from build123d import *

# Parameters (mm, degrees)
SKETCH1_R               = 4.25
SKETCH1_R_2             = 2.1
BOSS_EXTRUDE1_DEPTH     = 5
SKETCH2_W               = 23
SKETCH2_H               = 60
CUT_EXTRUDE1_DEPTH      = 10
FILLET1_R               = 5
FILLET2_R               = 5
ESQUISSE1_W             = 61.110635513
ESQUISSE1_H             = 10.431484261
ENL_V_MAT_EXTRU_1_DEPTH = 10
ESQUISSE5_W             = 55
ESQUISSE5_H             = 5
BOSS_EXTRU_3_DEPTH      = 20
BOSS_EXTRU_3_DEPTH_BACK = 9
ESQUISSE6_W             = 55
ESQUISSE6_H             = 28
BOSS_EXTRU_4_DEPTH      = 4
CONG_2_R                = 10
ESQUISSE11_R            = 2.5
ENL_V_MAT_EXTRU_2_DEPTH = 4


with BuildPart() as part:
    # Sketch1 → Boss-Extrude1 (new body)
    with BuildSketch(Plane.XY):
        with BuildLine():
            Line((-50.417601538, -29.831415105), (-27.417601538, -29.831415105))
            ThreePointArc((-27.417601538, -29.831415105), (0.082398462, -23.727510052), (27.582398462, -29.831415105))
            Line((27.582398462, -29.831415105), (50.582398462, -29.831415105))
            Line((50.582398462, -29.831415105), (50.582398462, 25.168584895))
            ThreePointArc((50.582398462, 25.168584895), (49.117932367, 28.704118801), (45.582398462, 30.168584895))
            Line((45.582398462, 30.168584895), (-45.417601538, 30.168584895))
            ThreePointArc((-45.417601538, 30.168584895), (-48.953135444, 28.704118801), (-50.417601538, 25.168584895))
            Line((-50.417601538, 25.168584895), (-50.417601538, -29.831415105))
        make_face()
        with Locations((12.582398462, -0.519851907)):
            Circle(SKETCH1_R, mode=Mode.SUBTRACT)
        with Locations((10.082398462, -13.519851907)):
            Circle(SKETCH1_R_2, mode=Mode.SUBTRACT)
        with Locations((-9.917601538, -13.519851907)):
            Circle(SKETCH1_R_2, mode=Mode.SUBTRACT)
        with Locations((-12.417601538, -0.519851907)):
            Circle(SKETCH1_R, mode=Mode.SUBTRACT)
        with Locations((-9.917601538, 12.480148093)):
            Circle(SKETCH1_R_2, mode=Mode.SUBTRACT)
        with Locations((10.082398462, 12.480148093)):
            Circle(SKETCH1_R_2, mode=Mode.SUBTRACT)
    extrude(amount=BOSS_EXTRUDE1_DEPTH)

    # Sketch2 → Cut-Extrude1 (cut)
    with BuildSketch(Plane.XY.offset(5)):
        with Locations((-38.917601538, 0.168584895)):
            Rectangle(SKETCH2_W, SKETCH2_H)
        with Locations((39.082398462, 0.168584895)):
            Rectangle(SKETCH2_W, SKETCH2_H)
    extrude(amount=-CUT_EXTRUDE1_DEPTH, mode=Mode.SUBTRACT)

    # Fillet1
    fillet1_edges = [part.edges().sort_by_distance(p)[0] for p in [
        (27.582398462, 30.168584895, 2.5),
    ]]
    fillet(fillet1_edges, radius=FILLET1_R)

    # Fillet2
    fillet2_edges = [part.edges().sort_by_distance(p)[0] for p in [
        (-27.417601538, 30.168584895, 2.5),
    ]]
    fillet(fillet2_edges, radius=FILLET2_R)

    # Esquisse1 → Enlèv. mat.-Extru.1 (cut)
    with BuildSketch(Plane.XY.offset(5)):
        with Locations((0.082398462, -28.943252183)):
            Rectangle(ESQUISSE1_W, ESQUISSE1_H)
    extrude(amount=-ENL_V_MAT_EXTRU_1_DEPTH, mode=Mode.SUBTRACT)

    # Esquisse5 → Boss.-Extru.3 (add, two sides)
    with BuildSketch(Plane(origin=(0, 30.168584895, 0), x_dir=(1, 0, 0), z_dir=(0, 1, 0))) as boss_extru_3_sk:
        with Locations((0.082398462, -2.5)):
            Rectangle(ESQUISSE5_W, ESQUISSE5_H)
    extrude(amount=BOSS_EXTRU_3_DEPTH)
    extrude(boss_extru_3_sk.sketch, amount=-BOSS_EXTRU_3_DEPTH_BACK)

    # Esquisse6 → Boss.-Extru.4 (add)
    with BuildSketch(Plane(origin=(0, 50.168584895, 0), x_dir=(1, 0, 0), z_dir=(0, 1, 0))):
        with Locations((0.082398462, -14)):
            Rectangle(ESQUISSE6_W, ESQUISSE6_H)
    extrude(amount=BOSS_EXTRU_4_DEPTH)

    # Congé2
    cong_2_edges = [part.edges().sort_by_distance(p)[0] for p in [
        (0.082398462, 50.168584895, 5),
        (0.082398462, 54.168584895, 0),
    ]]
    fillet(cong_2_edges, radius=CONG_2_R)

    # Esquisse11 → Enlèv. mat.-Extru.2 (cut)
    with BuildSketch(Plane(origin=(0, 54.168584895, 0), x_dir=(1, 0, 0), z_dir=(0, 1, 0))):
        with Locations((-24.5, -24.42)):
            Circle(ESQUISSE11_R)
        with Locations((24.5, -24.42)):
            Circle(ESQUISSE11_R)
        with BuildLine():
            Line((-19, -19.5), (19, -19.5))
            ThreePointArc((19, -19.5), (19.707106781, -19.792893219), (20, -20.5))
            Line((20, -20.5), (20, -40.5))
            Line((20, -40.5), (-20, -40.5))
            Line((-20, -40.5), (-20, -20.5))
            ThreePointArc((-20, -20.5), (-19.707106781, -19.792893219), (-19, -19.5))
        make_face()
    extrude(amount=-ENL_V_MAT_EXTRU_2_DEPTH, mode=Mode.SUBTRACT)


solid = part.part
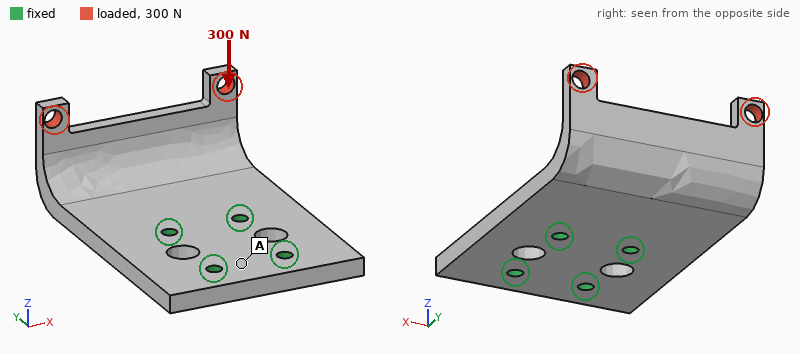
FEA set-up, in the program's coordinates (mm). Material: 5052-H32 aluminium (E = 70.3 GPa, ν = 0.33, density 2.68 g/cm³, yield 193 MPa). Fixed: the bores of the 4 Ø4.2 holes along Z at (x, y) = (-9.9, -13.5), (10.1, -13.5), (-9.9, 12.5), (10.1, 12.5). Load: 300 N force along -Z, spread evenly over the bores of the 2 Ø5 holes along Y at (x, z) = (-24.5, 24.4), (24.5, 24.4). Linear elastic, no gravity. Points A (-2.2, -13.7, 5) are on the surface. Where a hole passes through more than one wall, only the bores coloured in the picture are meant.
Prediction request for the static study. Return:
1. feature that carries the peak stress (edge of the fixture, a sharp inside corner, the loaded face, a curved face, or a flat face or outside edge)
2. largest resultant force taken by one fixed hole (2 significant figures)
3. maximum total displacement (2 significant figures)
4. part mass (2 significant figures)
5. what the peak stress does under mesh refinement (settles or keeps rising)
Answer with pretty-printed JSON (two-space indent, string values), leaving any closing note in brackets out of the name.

{
  "feature that carries the peak stress": "edge of the fixture",
  "largest resultant force taken by one fixed hole": "220 N",
  "maximum total displacement": "0.23 mm",
  "part mass": "65 g",
  "what the peak stress does under mesh refinement": "keeps rising"
}
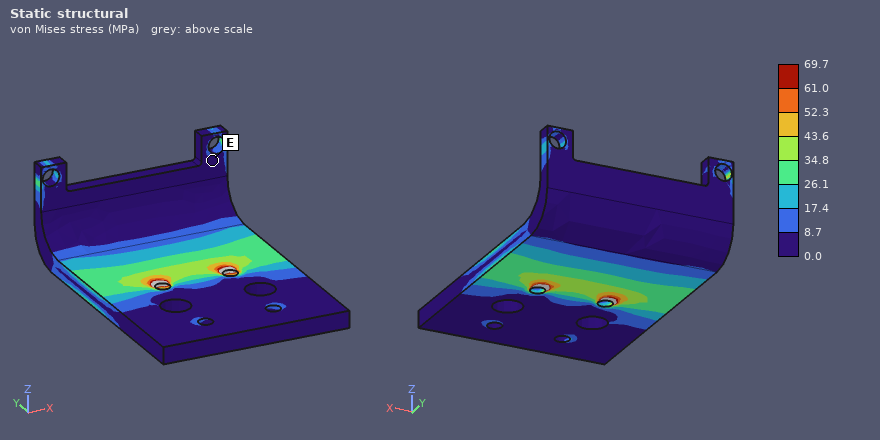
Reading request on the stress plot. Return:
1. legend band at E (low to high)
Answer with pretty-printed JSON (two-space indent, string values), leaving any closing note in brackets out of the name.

{
  "legend band at E": "0.0 to 8.7 MPa"
}
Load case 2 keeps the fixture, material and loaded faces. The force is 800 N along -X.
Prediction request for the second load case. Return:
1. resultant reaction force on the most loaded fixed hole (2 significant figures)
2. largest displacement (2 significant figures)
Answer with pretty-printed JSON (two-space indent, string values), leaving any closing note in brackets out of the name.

{
  "resultant reaction force on the most loaded fixed hole": "1.1 kN",
  "largest displacement": "0.31 mm"
}
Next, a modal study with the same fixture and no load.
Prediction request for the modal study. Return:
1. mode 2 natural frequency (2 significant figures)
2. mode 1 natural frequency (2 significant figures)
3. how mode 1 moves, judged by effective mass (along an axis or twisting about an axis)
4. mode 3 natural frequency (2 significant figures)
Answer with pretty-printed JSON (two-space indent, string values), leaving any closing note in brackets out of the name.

{
  "mode 2 natural frequency": "2900 Hz",
  "mode 1 natural frequency": "1600 Hz",
  "how mode 1 moves, judged by effective mass": "along Z",
  "mode 3 natural frequency": "7300 Hz"
}
